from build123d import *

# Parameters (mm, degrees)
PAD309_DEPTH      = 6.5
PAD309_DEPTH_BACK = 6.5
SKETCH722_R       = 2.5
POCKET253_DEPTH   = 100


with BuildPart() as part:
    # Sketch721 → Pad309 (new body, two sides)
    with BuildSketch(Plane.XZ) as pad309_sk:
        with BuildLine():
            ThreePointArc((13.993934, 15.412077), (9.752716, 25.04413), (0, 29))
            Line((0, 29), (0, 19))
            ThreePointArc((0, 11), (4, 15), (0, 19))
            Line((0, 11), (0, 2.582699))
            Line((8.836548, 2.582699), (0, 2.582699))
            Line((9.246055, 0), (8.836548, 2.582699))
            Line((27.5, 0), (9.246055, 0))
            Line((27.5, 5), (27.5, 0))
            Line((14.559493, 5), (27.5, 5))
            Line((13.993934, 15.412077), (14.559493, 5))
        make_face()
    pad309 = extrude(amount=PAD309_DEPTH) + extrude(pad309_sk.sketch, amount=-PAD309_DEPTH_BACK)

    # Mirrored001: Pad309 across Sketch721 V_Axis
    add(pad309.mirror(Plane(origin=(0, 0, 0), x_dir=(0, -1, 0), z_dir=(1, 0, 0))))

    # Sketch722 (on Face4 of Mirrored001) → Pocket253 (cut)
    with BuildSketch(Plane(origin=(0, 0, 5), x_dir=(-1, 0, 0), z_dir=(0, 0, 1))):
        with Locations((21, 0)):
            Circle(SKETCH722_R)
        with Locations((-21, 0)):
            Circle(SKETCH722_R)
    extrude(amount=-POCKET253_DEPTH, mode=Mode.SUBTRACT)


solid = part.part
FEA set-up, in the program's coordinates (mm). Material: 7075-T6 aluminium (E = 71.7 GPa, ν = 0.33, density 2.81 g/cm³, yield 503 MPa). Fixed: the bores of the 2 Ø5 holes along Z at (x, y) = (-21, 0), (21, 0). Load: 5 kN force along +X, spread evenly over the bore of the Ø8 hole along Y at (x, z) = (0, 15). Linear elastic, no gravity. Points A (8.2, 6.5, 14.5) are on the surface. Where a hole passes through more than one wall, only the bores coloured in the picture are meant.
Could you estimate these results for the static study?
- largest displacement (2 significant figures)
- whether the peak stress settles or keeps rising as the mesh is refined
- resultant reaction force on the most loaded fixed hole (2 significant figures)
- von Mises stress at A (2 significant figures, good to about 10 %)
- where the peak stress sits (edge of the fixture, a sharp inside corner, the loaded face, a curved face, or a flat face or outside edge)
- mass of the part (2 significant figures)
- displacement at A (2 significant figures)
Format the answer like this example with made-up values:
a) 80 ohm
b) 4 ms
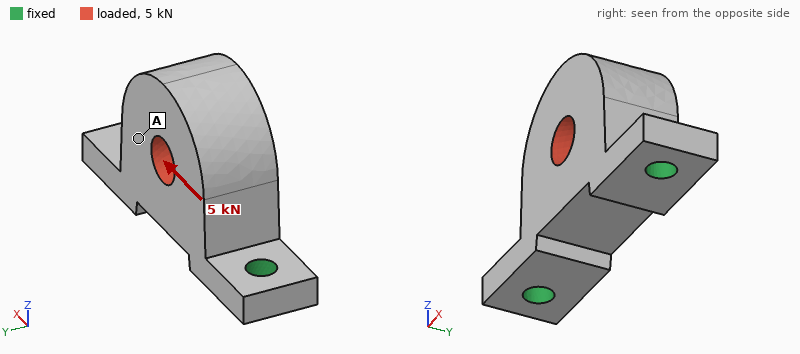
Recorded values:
a) 36 µm
b) keeps rising
c) 3.1 kN
d) 29 MPa
e) edge of the fixture
f) 28 g
g) 22 µm
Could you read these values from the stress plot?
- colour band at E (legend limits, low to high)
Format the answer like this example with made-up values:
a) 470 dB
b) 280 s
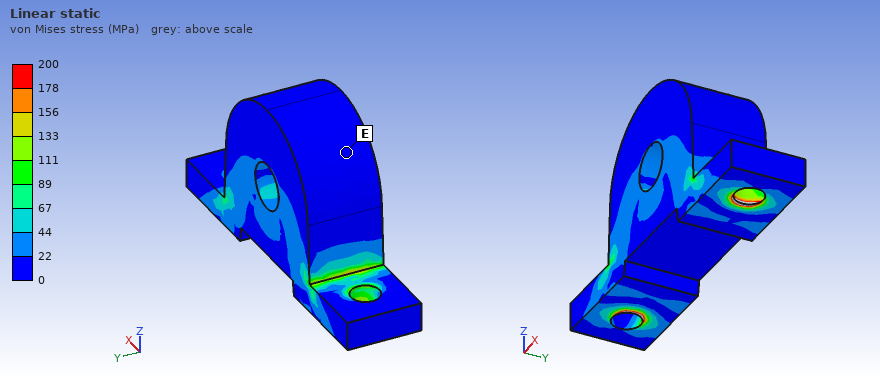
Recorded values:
a) 0 to 22 MPa
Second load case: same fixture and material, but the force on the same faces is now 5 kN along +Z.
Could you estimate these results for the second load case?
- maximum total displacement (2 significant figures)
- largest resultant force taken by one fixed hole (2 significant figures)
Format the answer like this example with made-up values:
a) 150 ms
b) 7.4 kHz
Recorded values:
a) 31 µm
b) 3.1 kN
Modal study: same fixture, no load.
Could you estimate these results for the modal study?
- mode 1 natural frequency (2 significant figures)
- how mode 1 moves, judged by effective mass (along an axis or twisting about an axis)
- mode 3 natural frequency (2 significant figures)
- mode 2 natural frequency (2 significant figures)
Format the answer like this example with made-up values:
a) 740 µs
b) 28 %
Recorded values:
a) 4400 Hz
b) along Y
c) 14 kHz
d) 14 kHz
